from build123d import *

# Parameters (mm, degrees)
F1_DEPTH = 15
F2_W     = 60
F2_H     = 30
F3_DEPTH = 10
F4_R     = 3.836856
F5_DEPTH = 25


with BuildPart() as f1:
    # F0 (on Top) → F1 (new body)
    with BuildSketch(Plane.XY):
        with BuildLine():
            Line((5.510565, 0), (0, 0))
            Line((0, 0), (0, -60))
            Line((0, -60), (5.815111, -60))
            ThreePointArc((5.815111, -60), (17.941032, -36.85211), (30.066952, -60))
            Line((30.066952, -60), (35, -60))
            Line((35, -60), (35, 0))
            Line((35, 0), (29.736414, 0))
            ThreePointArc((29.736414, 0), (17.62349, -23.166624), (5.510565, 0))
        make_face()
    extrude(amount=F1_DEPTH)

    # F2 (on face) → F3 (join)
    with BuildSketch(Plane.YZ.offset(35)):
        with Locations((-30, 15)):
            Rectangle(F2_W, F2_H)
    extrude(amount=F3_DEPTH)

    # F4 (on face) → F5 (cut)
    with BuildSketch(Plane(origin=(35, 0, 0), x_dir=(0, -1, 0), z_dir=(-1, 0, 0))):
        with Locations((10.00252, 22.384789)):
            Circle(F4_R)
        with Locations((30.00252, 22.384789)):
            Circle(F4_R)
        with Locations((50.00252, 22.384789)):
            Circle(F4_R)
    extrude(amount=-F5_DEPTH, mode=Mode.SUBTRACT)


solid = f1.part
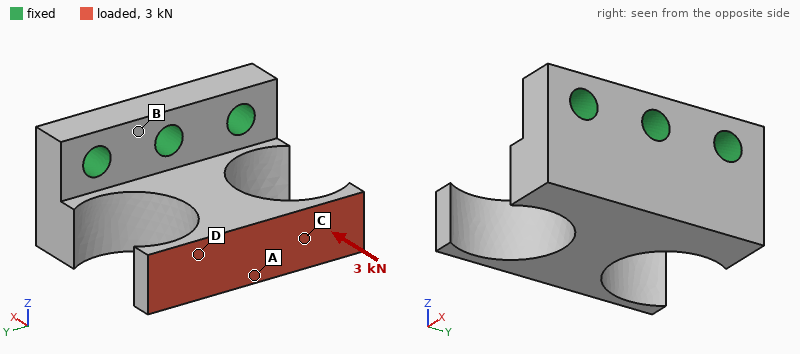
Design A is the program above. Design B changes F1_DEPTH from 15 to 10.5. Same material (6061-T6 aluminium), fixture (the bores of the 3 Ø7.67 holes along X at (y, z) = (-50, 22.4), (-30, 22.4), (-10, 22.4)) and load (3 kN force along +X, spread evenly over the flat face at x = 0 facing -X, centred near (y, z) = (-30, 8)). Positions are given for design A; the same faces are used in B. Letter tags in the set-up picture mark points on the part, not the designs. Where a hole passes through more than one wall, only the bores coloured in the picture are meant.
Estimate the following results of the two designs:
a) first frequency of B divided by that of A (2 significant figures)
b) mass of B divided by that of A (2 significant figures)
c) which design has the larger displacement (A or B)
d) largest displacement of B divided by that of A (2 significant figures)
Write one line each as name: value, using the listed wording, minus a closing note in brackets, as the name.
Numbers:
first frequency of B divided by that of A: 0.87
mass of B divided by that of A: 0.86
which design has the larger displacement: B
largest displacement of B divided by that of A: 1.4
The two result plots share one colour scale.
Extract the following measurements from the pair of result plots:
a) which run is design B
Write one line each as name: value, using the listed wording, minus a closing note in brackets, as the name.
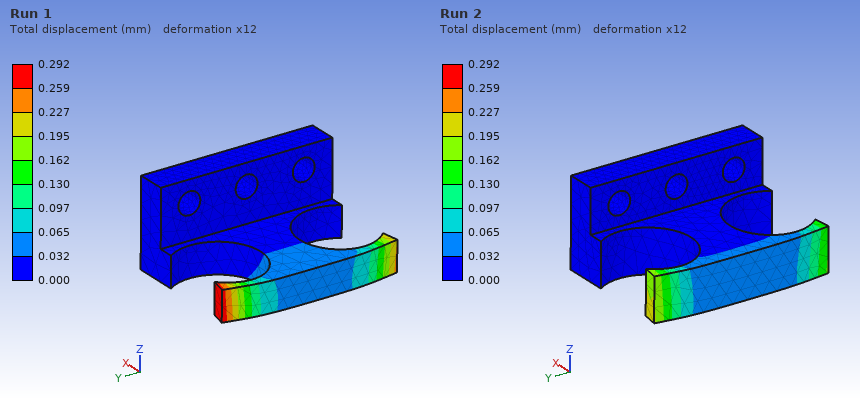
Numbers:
which run is design B: Run 1
